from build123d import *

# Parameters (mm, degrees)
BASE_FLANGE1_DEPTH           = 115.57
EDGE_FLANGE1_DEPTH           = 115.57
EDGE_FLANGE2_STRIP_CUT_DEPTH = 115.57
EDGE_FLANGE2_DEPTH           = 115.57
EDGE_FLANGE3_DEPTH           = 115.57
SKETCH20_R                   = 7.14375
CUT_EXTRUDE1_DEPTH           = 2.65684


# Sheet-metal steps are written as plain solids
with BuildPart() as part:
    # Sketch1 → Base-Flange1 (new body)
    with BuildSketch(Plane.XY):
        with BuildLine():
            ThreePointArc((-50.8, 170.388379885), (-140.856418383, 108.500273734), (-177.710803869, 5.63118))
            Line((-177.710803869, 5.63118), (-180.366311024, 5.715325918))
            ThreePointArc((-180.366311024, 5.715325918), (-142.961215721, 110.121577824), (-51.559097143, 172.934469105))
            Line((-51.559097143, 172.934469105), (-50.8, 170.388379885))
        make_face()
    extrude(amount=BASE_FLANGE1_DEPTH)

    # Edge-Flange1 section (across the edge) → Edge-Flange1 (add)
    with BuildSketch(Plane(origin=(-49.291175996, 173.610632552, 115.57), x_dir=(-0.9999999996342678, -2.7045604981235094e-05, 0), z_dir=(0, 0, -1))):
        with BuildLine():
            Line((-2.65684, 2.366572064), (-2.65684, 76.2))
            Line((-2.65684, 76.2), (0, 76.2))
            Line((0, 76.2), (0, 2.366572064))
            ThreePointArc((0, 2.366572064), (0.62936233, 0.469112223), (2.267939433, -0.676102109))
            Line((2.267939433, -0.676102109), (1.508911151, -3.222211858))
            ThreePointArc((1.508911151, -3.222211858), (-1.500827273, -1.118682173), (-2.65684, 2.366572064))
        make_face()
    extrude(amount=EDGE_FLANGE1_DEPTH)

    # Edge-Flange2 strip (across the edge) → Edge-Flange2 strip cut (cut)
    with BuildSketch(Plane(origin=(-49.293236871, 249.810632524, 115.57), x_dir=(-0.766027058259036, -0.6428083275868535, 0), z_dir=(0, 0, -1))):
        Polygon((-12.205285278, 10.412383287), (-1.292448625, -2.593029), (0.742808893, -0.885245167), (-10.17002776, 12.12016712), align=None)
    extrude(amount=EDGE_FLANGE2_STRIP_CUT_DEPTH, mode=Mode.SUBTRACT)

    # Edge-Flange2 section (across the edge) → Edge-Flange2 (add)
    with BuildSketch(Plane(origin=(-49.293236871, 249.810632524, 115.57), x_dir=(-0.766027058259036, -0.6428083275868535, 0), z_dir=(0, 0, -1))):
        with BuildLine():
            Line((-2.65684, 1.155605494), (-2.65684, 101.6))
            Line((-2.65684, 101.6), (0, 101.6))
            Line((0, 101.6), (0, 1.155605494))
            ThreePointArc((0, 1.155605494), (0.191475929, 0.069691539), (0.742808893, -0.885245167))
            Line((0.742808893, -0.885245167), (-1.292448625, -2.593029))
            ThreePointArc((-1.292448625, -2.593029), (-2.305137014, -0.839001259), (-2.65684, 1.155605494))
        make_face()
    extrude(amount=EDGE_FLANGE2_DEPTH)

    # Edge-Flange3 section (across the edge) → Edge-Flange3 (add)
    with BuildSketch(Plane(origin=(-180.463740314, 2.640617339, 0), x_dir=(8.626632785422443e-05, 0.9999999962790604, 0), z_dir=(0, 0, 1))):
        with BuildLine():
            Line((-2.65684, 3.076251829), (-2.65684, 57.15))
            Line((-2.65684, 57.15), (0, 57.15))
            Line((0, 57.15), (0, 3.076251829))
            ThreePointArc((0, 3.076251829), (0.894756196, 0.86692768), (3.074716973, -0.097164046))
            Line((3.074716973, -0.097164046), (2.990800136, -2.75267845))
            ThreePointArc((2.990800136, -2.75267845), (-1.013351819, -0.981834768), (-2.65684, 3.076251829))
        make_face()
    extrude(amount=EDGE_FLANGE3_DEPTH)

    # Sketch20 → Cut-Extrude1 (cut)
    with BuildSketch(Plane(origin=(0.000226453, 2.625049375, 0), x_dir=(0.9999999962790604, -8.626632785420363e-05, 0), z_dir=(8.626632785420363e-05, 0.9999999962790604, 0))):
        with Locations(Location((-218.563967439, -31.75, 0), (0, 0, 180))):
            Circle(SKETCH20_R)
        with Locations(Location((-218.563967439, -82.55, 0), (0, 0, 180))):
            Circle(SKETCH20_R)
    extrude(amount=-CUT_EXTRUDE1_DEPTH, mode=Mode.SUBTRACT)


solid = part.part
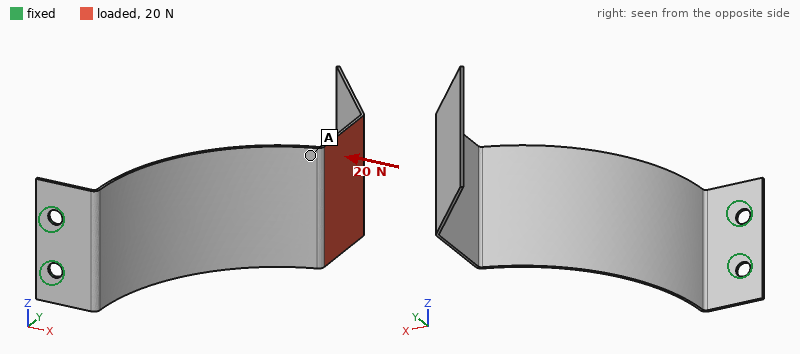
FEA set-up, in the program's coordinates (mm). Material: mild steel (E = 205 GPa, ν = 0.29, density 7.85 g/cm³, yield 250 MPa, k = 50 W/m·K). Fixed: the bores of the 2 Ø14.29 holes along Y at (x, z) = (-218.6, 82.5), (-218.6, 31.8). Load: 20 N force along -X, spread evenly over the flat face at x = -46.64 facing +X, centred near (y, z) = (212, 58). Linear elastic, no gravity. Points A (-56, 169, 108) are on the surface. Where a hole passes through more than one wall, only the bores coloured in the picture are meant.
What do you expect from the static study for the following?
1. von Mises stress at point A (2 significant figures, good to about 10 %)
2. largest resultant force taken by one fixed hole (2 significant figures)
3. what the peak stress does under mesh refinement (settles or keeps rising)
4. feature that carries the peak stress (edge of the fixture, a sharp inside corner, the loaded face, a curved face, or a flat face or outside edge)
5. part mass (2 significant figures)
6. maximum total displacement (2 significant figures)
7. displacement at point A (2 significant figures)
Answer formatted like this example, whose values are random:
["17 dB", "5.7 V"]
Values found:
["5.6 MPa", "12 N", "keeps rising", "edge of the fixture", "1.1 kg", "4.6 mm", "2.5 mm"]
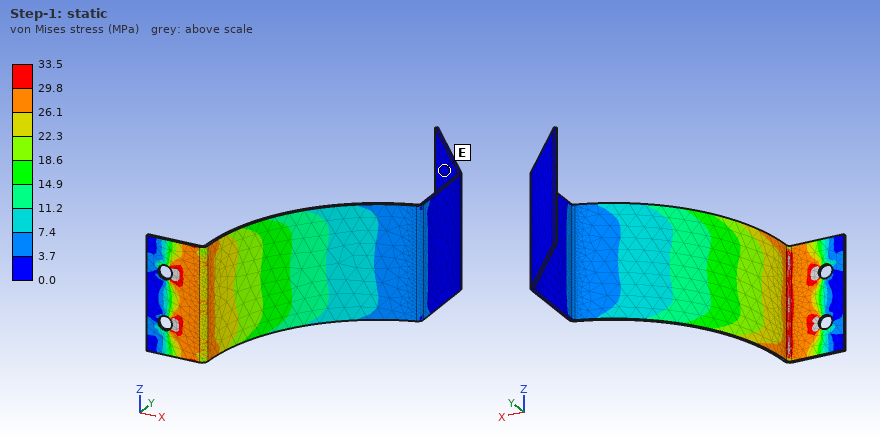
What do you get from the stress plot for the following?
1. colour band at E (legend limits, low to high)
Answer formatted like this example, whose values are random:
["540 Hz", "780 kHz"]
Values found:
["0.0 to 3.7 MPa"]
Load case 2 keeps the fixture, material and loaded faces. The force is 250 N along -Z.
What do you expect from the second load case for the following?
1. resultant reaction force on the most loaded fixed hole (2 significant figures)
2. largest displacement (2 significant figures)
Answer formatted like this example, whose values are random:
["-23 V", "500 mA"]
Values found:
["1.0 kN", "3.1 mm"]
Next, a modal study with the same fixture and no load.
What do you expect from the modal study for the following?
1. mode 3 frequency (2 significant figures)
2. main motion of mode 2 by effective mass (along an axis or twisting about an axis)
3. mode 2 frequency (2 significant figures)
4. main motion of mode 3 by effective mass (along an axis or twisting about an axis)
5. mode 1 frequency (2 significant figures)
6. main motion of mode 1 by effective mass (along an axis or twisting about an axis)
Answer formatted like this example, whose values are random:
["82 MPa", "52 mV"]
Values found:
["66 Hz", "along Z", "47 Hz", "along Y", "13 Hz", "along X"]
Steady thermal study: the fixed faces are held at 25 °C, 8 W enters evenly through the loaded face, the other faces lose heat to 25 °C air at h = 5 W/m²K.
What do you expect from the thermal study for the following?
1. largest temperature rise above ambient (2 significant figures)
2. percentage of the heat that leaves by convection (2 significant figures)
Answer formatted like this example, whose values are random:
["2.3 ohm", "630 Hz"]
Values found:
["32 K", "92 %"]
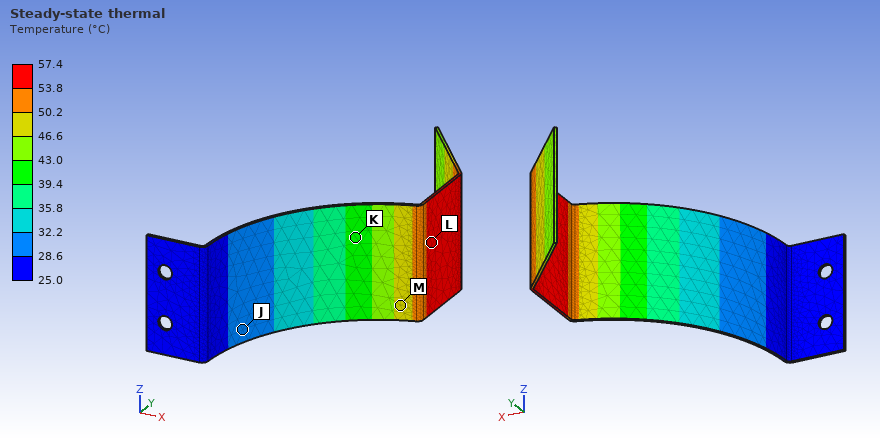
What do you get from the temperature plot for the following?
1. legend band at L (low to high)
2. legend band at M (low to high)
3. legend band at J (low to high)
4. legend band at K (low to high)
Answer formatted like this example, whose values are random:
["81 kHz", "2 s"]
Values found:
["53.8 to 57.4 °C", "46.6 to 50.2 °C", "28.6 to 32.2 °C", "39.4 to 43.0 °C"]
